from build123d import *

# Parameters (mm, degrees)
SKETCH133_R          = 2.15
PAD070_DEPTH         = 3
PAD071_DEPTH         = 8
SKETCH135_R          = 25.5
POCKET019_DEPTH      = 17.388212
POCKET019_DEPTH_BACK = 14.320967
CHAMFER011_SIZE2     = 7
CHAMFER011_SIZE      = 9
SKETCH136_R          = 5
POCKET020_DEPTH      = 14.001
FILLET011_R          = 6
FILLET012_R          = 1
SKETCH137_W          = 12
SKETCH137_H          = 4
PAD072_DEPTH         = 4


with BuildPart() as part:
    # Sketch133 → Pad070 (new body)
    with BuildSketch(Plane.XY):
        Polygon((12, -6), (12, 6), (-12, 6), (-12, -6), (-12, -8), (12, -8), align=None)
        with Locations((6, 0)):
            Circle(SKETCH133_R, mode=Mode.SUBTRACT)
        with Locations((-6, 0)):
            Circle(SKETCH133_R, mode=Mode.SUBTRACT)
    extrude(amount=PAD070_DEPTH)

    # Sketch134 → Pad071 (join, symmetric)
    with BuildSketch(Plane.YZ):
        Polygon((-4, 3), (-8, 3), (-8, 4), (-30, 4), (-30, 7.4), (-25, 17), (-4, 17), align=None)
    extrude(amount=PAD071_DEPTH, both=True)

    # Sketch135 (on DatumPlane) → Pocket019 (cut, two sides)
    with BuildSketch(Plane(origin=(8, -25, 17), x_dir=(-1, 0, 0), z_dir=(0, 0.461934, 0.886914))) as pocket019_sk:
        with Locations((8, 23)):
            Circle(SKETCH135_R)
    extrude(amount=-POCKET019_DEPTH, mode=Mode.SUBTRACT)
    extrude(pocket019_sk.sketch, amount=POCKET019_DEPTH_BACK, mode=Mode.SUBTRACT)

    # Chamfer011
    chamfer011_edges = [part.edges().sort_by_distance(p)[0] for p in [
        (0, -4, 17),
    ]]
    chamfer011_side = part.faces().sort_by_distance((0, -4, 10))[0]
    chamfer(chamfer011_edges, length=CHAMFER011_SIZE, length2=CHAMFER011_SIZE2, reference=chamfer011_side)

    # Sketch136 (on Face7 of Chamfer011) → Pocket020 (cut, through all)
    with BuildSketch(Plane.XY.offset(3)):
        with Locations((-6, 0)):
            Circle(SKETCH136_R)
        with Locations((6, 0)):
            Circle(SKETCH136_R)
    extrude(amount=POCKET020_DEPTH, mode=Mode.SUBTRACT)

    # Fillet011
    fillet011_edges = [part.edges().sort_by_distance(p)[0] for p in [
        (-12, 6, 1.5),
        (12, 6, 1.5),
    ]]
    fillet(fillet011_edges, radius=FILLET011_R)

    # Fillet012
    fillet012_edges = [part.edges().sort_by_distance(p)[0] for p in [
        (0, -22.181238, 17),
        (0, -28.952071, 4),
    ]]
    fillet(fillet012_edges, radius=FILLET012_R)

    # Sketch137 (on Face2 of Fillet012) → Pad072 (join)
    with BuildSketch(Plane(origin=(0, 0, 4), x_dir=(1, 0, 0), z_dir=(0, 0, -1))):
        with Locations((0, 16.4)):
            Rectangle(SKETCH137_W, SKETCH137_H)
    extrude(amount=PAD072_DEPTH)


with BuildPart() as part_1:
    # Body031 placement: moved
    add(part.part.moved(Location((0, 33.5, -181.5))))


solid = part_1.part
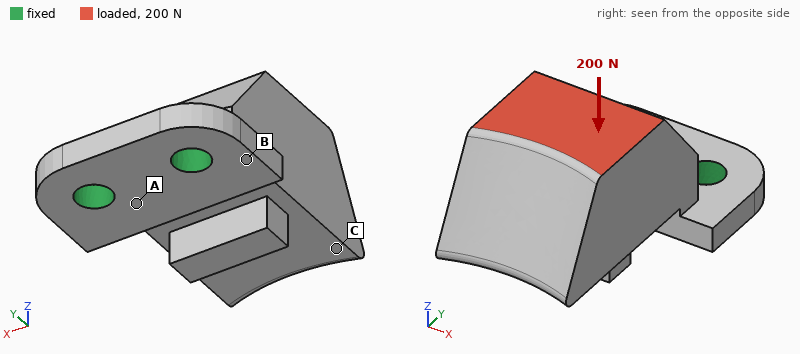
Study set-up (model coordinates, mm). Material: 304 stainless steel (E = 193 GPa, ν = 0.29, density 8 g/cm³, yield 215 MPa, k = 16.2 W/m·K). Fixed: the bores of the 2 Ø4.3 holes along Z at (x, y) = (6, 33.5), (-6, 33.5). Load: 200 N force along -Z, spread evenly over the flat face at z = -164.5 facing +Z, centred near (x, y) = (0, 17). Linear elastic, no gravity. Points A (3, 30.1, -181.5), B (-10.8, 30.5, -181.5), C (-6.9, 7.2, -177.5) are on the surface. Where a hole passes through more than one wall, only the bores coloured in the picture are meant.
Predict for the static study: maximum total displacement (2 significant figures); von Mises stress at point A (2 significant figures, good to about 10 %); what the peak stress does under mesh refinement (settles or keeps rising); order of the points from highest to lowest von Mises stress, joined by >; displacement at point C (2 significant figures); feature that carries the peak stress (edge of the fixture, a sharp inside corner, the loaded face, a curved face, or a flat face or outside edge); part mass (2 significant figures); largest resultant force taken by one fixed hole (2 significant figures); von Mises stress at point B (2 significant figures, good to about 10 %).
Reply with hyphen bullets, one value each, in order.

- 48 µm
- 70 MPa
- keeps rising
- A > B > C
- 41 µm
- edge of the fixture
- 41 g
- 100 N
- 42 MPa
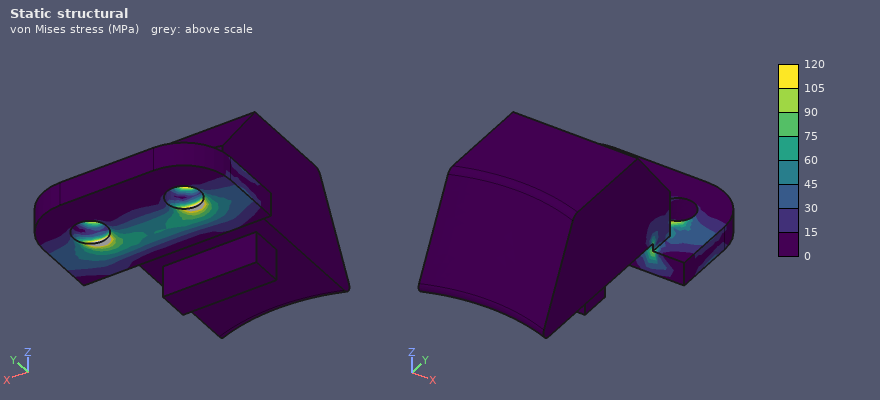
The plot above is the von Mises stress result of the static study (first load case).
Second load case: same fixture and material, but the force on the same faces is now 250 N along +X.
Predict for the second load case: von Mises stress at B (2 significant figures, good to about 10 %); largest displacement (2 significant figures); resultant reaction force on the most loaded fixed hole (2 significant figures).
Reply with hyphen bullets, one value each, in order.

- 13 MPa
- 7.4 µm
- 420 N
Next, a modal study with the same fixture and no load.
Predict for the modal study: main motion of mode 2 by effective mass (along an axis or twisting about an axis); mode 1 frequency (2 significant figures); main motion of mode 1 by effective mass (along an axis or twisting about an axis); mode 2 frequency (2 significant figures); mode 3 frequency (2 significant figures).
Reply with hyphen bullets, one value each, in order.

- along X
- 2000 Hz
- along Z
- 6900 Hz
- 10 kHz
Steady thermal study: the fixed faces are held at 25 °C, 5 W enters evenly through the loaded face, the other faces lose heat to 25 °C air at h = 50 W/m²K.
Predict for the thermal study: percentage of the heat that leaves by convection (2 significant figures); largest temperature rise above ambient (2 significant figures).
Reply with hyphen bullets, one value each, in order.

- 49 %
- 42 K
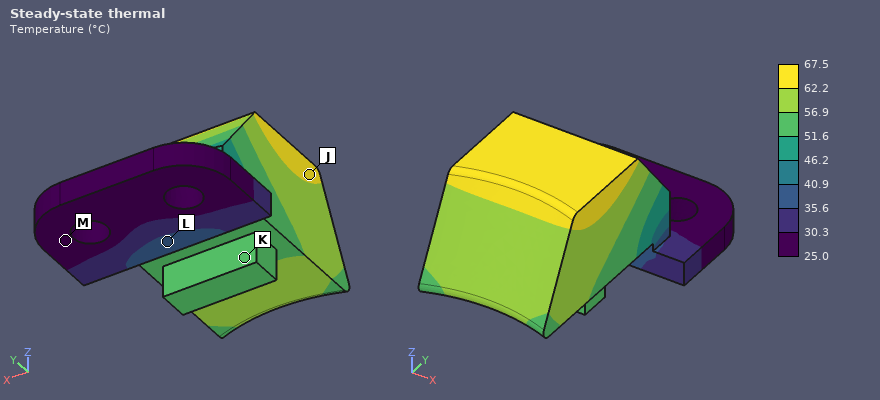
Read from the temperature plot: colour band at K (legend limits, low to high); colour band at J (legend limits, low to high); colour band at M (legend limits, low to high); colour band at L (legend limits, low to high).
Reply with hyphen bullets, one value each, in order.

- 51.6 to 56.9 °C
- 62.2 to 67.5 °C
- 25.0 to 30.3 °C
- 35.6 to 40.9 °C
